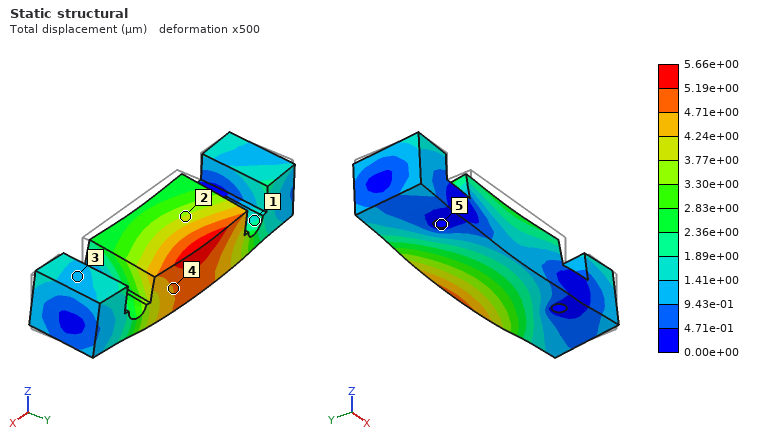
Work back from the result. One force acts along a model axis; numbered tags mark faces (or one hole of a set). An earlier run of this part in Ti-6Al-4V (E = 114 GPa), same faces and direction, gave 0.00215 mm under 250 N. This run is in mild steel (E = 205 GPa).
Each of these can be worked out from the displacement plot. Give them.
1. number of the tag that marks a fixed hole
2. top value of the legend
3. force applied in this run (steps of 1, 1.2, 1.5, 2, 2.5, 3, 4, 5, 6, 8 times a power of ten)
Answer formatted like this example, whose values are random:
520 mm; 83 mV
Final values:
5; 5.66e+00 µm; 1.2 kN
